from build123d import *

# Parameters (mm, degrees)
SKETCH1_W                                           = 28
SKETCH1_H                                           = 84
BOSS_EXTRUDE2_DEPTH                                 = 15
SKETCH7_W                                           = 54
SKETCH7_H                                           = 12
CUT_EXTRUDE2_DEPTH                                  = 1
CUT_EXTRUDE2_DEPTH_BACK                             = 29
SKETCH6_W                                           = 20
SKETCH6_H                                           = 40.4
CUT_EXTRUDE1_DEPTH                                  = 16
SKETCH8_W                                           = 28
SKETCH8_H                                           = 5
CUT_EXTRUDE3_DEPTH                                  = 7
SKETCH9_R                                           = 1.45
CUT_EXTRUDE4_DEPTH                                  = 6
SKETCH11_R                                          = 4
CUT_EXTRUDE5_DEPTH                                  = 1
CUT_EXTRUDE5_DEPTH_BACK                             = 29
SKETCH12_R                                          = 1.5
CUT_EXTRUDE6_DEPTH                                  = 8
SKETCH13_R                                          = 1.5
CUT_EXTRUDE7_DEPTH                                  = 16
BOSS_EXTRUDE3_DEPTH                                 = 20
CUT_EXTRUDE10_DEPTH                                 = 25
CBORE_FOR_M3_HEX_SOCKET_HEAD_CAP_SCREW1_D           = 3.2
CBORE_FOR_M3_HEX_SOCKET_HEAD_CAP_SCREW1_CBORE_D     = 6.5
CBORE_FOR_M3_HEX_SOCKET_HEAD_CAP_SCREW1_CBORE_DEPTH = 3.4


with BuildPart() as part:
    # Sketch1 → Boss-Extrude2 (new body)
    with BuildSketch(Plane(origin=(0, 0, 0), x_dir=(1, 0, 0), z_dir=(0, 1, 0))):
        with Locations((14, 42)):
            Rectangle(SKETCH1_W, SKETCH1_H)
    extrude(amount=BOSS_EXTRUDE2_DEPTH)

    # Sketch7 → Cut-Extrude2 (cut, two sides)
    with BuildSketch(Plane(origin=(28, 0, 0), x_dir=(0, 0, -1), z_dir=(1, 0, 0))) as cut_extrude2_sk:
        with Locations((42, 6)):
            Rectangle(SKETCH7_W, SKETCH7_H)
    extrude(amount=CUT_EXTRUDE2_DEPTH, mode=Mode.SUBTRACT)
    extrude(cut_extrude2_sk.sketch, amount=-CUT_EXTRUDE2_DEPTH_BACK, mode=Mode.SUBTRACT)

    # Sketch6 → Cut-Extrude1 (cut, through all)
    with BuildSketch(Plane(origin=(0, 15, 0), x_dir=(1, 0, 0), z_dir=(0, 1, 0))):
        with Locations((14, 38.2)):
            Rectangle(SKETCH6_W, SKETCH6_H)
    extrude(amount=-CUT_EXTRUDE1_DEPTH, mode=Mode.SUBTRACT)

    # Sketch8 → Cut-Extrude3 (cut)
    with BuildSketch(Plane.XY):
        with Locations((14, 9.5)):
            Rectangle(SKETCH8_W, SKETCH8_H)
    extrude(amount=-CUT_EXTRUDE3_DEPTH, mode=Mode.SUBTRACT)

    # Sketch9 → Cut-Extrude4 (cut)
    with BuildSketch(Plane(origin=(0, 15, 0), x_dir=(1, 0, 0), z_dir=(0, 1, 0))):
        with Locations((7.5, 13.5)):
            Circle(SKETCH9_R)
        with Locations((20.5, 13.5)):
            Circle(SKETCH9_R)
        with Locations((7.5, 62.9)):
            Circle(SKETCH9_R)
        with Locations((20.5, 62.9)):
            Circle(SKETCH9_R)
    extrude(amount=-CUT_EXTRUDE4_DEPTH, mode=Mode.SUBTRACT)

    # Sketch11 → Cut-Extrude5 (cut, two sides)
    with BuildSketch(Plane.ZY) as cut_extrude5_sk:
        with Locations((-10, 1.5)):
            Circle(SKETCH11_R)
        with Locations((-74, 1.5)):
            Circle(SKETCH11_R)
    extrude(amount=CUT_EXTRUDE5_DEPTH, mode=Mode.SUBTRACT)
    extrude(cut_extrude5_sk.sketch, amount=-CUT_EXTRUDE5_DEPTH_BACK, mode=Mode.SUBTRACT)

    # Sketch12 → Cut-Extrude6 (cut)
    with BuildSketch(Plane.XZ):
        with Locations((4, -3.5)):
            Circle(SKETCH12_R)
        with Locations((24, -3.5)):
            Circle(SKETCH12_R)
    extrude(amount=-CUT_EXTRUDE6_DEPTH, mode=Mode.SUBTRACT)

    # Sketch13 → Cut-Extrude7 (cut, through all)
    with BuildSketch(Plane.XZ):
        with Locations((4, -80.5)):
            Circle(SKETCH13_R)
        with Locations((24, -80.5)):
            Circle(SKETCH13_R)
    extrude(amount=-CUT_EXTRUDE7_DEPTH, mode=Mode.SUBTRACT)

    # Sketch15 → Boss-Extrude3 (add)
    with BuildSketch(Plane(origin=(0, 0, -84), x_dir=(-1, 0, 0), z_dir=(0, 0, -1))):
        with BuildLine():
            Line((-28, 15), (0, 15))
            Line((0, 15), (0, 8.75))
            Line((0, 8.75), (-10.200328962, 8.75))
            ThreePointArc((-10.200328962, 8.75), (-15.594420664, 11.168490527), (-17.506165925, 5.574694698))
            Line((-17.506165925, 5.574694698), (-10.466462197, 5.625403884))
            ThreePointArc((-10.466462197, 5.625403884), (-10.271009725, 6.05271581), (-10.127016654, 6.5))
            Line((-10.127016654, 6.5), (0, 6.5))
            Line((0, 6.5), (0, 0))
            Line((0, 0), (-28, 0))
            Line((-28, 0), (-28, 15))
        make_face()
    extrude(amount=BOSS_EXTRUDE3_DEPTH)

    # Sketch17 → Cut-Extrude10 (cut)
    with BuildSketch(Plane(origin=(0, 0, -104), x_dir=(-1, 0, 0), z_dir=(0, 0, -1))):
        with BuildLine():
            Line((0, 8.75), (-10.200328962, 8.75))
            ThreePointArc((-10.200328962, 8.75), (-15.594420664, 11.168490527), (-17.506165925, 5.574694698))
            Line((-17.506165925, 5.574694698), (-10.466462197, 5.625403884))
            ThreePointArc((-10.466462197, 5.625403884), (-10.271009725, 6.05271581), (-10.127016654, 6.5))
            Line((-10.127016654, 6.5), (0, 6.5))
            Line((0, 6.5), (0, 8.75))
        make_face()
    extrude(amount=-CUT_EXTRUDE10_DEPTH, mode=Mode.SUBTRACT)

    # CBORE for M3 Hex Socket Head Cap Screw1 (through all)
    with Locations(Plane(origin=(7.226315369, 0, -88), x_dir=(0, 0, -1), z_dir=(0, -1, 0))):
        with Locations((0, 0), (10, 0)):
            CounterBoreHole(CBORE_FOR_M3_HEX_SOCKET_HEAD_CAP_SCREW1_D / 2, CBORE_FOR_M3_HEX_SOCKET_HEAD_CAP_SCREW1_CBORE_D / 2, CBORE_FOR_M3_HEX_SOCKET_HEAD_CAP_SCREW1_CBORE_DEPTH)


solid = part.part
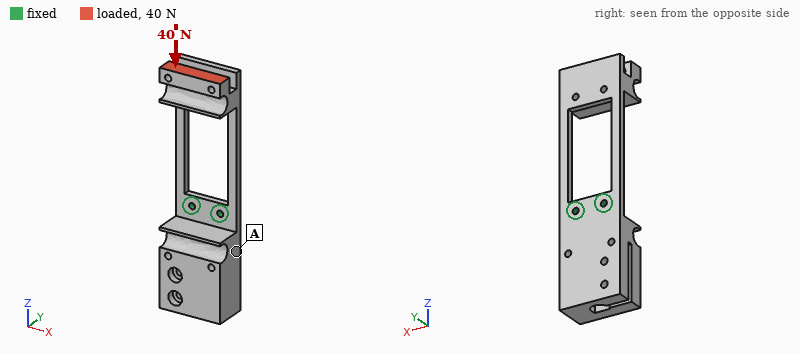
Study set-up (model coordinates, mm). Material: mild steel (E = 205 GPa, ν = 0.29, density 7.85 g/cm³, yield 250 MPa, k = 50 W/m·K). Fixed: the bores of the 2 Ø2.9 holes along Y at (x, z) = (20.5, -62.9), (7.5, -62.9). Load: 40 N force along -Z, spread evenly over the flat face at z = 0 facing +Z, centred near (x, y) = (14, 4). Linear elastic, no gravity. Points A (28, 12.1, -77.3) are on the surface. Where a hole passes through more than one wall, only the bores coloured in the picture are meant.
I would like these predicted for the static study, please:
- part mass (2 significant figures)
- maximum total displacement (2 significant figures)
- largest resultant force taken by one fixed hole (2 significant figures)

140 g
0.21 mm
20 N
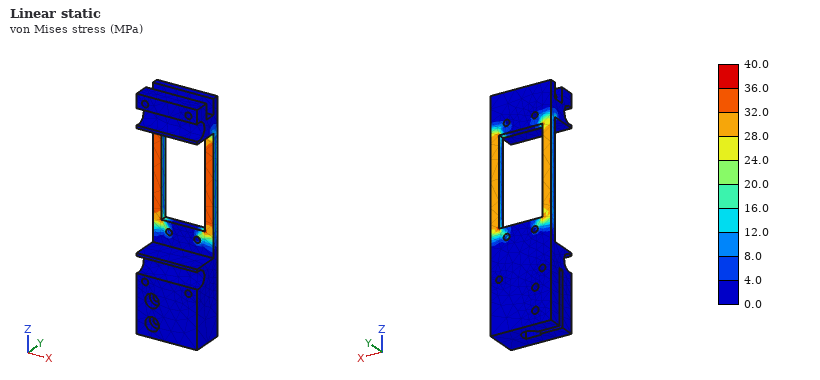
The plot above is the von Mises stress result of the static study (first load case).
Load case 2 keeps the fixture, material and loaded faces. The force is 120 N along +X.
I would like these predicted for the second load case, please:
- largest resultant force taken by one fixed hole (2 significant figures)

450 N
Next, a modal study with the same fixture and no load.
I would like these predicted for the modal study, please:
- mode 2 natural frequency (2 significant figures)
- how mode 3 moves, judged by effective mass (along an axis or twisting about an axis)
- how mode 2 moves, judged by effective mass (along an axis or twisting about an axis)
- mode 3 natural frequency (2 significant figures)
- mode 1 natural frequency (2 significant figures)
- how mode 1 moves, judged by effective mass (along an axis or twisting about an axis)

660 Hz
along Y
along X
920 Hz
220 Hz
along Y
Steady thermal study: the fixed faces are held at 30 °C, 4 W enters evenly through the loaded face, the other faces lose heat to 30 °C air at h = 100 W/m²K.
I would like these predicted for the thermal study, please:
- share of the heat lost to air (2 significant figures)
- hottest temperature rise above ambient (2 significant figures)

97 %
18 K
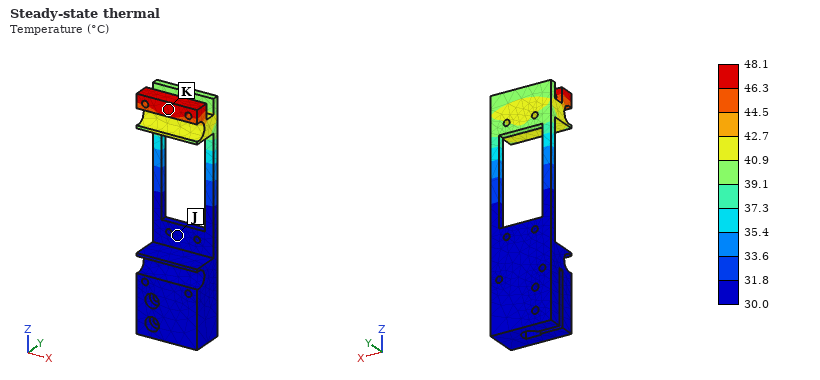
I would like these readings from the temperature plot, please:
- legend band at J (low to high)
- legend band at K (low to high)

30.0 to 31.8 °C
46.3 to 48.1 °C
